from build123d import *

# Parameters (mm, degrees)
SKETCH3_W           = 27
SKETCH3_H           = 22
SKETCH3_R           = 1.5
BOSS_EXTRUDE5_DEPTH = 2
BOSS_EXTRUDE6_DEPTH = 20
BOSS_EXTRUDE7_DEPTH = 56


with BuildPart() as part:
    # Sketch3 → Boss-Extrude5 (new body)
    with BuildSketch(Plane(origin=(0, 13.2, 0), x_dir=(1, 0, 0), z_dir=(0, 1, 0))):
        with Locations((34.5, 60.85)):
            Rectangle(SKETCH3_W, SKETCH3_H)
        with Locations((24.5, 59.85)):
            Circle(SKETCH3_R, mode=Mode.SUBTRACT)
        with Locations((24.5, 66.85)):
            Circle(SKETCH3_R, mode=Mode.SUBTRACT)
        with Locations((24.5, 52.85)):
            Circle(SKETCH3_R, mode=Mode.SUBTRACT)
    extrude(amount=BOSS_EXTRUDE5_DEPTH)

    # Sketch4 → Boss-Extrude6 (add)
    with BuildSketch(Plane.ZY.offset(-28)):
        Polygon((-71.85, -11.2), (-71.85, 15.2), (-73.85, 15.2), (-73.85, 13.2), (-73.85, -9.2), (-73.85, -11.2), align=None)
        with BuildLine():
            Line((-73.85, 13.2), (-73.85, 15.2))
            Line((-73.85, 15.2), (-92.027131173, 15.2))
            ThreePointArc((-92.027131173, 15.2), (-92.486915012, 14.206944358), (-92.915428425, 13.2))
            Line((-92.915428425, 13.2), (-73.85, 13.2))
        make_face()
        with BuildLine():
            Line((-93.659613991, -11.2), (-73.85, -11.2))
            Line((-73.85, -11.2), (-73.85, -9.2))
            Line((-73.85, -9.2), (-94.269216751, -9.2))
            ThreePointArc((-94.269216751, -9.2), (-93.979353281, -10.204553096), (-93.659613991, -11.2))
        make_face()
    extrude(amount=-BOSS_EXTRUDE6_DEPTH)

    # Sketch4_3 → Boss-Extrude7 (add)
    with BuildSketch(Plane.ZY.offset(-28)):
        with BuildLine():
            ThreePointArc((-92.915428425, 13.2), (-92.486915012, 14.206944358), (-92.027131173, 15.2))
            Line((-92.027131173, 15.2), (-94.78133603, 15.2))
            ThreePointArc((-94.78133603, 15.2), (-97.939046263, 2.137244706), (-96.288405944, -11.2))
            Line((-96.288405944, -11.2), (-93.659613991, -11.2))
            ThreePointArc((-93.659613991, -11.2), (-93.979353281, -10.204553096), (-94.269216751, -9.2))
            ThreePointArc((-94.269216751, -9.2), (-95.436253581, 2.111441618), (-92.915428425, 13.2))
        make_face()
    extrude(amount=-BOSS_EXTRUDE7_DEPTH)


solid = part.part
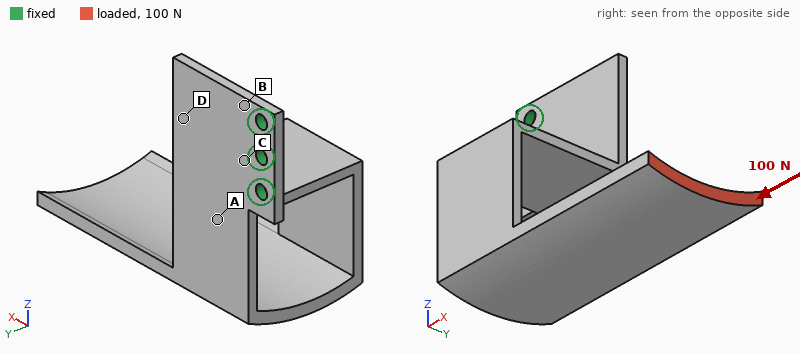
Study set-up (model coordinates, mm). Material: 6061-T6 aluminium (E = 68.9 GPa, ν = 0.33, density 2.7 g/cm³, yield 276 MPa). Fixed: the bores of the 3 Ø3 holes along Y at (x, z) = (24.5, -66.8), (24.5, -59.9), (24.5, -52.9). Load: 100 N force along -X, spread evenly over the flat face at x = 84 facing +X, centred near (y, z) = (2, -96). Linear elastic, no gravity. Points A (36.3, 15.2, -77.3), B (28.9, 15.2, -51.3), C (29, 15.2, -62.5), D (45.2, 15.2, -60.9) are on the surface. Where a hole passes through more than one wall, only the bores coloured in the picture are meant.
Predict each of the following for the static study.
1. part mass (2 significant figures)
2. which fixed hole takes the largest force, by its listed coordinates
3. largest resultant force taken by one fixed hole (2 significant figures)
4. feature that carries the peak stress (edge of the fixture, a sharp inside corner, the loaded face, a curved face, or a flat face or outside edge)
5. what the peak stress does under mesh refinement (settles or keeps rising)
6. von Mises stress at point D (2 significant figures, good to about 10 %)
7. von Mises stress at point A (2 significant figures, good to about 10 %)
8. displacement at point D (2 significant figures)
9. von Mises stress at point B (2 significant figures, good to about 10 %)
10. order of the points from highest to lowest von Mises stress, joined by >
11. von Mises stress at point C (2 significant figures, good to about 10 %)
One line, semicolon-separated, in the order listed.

20 g; (24.5, -66.8); 290 N; a sharp inside corner; keeps rising; 25 MPa; 10 MPa; 0.13 mm; 57 MPa; C > B > D > A; 69 MPa
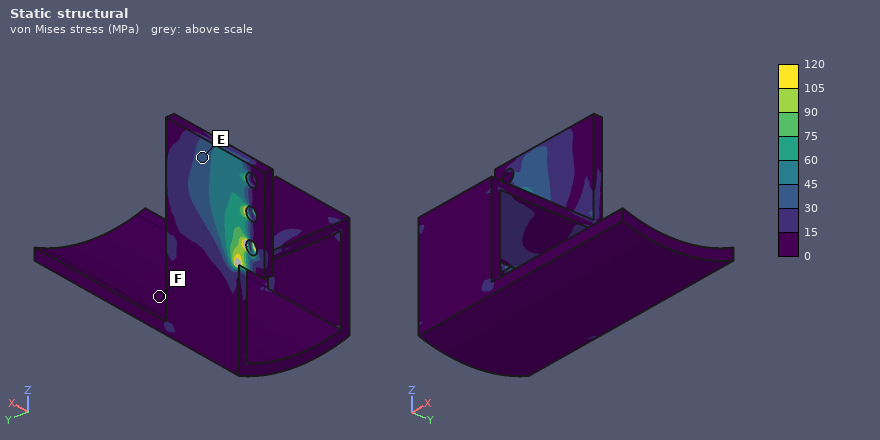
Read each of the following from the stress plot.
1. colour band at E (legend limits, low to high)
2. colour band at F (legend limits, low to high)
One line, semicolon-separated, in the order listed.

30 to 45 MPa; 0 to 15 MPa
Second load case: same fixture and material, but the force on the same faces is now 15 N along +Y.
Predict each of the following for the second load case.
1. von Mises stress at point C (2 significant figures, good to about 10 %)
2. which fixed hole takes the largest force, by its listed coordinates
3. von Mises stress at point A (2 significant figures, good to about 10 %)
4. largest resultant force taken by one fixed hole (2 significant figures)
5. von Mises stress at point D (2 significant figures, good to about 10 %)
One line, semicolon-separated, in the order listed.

52 MPa; (24.5, -66.8); 14 MPa; 37 N; 24 MPa
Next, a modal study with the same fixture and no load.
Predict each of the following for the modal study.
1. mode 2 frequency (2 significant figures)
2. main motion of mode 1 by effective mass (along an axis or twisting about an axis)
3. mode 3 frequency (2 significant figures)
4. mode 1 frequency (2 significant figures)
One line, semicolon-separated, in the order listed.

670 Hz; along Y; 1500 Hz; 290 Hz
